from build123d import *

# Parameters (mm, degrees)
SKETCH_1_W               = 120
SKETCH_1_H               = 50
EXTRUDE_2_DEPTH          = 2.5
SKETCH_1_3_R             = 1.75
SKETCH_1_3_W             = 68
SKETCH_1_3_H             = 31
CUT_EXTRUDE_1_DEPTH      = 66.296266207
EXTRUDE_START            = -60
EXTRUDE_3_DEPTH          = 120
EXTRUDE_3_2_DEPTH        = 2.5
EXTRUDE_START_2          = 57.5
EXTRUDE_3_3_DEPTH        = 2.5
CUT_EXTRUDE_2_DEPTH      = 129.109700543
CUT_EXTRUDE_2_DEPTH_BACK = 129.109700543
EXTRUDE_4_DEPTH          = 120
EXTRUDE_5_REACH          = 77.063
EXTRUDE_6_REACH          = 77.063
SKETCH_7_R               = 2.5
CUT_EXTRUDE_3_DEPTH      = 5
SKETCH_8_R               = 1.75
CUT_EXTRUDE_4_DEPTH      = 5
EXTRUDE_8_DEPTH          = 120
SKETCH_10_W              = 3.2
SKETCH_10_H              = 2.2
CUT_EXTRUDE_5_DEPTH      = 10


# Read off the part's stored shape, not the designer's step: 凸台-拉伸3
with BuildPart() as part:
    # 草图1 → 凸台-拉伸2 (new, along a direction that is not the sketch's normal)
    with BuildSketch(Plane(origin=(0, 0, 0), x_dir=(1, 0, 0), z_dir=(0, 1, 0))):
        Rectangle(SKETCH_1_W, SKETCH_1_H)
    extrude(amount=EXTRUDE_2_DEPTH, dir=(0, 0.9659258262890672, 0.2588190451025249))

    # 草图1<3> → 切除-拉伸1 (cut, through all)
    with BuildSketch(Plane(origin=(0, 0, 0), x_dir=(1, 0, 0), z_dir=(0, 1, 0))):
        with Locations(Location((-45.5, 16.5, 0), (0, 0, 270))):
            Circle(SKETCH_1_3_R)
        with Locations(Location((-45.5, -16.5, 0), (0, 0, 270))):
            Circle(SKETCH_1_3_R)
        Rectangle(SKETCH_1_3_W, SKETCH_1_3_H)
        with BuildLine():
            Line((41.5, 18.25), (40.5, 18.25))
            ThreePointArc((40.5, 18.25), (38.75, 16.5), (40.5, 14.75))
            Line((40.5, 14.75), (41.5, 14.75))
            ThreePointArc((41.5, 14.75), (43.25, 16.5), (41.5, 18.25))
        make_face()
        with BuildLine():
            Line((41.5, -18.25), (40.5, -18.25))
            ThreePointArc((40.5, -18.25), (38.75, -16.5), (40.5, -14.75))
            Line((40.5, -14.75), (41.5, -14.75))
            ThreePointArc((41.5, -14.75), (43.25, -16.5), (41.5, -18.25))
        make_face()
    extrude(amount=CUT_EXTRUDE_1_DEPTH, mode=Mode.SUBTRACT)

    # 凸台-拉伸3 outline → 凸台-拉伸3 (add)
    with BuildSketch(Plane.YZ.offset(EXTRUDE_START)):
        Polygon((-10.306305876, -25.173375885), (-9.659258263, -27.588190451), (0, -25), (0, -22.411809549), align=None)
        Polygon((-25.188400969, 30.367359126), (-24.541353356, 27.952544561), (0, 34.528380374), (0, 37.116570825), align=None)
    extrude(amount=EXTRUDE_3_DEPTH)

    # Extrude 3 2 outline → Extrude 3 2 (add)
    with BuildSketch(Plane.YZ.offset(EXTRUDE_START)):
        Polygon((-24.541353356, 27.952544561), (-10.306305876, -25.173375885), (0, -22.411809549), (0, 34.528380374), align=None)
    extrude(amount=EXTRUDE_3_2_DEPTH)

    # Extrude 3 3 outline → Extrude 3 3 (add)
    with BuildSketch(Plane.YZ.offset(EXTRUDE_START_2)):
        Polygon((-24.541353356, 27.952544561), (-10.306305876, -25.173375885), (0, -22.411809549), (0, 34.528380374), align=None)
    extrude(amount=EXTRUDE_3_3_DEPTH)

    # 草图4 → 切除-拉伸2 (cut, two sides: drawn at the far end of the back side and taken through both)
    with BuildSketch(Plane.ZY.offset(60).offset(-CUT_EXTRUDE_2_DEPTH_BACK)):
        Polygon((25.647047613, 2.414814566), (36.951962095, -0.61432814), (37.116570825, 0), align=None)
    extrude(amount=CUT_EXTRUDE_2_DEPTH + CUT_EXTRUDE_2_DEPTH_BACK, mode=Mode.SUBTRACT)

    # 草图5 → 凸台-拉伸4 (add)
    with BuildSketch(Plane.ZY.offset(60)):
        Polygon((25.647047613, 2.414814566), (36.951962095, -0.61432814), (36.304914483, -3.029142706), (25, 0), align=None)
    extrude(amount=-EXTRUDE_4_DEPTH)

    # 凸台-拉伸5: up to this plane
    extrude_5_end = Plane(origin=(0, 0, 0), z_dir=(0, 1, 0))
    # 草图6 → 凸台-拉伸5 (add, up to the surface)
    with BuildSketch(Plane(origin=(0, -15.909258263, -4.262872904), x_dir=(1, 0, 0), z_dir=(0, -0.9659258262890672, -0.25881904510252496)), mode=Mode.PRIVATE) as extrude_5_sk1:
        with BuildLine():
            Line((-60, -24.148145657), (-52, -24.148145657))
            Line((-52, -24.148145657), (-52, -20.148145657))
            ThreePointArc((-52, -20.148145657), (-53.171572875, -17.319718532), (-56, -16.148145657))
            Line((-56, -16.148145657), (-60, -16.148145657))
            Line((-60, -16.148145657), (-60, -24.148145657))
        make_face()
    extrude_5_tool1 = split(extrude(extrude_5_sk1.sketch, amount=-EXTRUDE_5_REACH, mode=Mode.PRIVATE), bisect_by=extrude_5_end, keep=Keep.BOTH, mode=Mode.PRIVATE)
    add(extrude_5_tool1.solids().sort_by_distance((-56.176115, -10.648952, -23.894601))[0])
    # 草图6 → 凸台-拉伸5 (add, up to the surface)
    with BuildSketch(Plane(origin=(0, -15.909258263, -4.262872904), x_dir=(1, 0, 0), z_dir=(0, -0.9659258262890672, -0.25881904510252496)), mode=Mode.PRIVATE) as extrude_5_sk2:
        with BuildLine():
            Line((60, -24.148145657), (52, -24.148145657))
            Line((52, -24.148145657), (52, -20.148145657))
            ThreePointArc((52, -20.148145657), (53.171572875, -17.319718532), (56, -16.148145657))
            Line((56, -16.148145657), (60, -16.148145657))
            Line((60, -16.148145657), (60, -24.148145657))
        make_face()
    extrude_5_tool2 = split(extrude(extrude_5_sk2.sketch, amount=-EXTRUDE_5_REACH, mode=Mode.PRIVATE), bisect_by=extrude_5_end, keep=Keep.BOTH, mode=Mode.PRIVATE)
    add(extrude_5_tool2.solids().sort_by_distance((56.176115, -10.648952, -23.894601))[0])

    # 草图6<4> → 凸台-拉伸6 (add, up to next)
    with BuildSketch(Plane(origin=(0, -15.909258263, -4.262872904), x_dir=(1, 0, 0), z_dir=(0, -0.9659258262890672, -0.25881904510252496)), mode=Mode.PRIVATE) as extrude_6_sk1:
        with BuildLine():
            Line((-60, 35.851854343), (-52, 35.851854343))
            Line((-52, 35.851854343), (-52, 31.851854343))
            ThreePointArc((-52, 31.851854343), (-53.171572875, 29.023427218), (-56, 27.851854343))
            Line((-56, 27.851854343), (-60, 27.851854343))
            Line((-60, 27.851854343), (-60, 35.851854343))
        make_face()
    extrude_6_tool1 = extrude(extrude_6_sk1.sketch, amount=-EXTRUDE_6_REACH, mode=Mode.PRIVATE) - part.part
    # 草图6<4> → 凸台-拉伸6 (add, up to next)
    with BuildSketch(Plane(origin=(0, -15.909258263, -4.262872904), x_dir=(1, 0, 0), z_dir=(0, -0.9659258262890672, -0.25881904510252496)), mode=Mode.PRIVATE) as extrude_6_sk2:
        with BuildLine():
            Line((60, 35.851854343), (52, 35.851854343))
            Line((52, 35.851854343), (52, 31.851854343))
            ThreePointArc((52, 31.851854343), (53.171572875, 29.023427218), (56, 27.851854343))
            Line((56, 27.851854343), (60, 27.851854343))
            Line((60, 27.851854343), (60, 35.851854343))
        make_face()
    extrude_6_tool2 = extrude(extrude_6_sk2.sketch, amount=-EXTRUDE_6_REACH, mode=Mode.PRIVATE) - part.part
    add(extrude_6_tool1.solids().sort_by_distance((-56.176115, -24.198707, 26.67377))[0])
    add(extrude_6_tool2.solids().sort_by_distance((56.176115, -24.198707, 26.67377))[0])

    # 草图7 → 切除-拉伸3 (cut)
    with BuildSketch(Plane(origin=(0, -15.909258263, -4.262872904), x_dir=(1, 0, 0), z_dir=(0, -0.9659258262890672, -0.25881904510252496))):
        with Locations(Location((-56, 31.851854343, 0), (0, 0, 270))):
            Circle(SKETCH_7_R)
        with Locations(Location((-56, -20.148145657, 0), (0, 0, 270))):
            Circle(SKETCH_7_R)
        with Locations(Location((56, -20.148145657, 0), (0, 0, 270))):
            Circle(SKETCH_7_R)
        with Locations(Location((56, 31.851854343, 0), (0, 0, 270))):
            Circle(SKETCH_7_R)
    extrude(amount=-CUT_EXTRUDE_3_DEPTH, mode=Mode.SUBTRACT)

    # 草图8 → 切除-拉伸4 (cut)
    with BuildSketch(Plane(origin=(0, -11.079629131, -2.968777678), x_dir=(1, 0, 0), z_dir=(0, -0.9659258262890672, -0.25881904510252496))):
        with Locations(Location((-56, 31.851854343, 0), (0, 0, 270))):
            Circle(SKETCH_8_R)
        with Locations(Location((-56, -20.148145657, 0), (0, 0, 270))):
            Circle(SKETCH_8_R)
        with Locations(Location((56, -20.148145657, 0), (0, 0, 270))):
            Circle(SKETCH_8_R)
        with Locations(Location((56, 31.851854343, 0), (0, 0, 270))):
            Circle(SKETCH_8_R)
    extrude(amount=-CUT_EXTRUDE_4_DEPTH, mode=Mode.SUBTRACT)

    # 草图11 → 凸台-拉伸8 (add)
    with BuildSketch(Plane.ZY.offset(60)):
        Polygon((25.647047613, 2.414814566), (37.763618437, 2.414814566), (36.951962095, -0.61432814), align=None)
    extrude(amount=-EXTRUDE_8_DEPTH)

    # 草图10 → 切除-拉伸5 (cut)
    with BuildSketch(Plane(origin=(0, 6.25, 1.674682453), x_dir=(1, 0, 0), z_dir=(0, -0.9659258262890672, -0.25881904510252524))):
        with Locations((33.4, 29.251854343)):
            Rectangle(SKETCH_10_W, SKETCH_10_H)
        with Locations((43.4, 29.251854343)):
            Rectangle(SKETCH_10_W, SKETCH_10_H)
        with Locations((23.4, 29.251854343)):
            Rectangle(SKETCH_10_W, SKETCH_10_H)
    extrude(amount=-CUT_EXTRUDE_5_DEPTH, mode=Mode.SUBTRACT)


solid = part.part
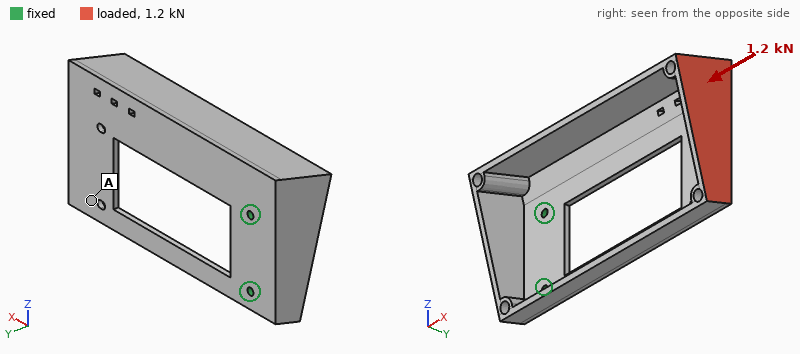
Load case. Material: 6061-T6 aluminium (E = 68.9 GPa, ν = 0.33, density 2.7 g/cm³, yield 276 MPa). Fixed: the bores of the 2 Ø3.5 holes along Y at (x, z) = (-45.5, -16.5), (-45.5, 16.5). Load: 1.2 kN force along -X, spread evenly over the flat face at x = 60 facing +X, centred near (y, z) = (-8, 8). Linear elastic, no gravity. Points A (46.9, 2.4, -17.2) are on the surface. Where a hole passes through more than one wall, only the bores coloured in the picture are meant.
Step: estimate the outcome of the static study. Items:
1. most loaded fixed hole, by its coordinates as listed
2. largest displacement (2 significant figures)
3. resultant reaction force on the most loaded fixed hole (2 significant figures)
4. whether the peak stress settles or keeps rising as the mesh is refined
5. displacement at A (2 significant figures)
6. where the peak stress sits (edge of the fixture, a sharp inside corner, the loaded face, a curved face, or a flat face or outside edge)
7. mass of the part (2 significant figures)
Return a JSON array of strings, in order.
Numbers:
["(-45.5, 16.5)", "1.5 mm", "880 N", "keeps rising", "0.99 mm", "edge of the fixture", "84 g"]
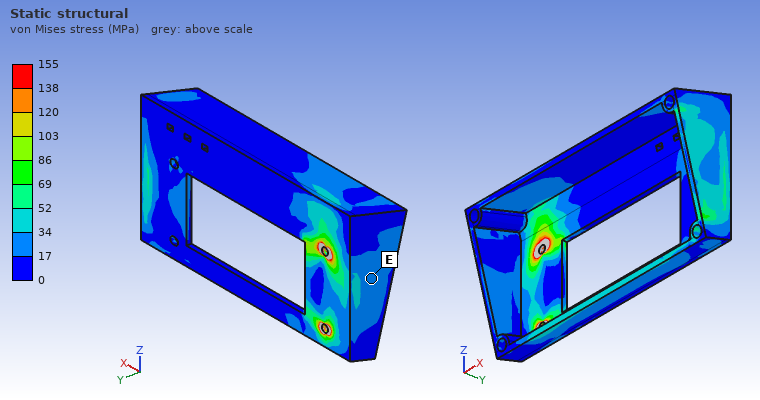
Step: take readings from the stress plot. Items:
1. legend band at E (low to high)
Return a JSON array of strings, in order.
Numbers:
["17 to 34 MPa"]
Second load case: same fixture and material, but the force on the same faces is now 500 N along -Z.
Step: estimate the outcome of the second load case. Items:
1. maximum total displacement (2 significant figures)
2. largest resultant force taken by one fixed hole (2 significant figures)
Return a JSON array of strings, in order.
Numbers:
["1.1 mm", "1.6 kN"]
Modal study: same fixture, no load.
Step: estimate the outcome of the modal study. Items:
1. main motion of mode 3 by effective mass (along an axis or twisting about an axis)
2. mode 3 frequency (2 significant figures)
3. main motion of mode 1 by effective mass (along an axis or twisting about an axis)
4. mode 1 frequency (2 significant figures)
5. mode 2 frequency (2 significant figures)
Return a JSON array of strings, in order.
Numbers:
["along Z", "1200 Hz", "along Y", "260 Hz", "600 Hz"]
